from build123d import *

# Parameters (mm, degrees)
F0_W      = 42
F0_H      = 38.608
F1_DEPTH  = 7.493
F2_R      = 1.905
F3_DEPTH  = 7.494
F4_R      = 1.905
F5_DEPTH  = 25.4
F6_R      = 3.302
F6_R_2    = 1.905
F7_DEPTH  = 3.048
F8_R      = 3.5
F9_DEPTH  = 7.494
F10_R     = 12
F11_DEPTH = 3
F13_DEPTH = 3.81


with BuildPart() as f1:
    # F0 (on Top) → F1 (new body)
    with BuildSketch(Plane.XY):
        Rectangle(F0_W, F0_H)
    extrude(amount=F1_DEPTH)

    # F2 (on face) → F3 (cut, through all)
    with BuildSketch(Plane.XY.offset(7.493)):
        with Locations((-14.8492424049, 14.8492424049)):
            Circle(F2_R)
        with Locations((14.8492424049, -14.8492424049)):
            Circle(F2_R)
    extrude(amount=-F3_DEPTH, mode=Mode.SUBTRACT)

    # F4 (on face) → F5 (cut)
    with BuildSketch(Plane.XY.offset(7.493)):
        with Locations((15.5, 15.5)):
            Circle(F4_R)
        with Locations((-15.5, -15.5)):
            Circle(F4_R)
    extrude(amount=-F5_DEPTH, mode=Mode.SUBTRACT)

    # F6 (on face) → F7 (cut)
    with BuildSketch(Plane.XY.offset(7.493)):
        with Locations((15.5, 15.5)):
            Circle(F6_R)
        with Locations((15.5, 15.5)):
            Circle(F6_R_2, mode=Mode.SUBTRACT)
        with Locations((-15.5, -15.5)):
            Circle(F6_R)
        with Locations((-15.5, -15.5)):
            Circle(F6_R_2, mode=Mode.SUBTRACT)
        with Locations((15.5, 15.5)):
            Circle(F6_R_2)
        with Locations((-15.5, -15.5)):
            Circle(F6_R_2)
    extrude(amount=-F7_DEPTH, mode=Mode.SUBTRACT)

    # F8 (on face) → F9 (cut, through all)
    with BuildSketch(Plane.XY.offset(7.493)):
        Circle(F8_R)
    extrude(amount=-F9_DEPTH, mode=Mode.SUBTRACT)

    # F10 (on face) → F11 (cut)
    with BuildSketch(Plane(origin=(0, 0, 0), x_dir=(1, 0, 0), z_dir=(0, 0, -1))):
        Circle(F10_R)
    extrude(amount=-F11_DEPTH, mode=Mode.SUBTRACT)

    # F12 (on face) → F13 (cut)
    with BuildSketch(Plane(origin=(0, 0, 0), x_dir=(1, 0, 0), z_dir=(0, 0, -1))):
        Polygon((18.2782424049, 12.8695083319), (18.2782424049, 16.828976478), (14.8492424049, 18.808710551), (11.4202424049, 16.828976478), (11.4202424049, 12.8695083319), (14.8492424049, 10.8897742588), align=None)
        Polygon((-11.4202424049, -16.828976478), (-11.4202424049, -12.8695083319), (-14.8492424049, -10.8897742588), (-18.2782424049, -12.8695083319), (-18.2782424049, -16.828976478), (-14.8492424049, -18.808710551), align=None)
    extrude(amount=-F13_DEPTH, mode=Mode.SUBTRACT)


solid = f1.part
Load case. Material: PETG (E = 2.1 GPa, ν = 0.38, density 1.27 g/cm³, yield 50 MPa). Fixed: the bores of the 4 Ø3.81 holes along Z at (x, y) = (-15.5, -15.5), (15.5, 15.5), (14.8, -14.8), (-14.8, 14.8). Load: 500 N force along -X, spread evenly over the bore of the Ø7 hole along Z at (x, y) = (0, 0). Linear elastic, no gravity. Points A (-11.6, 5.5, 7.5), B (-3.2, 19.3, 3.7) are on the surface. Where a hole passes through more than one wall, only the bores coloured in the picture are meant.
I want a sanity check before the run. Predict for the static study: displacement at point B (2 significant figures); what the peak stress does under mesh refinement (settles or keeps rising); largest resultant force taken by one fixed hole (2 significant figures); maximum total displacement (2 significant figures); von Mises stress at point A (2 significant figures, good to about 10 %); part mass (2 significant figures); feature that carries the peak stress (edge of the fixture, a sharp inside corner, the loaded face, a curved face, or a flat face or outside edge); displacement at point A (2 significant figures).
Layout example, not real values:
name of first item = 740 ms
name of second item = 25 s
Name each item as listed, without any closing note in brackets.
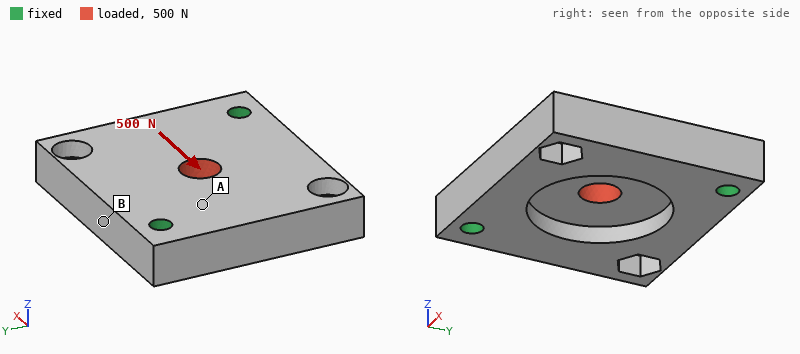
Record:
displacement at point B = 11 µm
what the peak stress does under mesh refinement = keeps rising
largest resultant force taken by one fixed hole = 140 N
maximum total displacement = 37 µm
von Mises stress at point A = 2.6 MPa
part mass = 13 g
feature that carries the peak stress = edge of the fixture
displacement at point A = 20 µm
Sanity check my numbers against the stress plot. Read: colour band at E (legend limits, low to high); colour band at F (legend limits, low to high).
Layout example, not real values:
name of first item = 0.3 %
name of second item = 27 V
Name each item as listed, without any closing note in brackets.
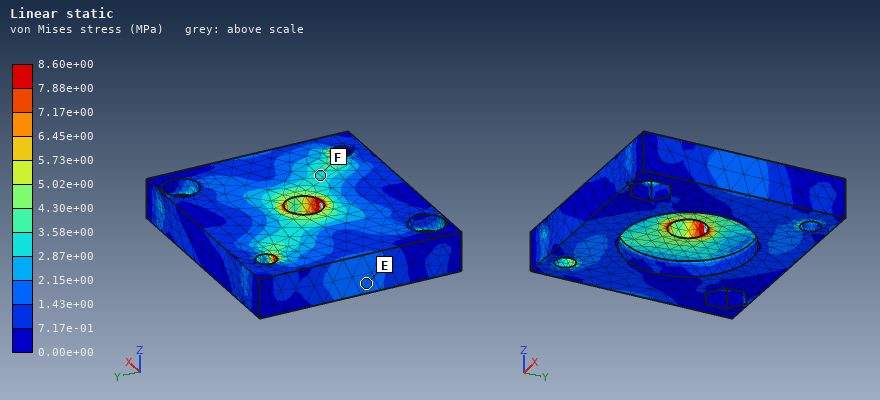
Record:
colour band at E = 1.43e+00 to 2.15e+00 MPa
colour band at F = 2.87e+00 to 3.58e+00 MPa
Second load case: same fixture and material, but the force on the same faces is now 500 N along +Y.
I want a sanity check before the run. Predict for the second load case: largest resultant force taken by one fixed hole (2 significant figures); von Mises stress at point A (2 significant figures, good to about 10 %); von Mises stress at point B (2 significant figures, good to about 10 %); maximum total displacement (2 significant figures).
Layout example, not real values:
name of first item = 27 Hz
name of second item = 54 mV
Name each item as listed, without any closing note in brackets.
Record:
largest resultant force taken by one fixed hole = 140 N
von Mises stress at point A = 2.1 MPa
von Mises stress at point B = 1.8 MPa
maximum total displacement = 38 µm
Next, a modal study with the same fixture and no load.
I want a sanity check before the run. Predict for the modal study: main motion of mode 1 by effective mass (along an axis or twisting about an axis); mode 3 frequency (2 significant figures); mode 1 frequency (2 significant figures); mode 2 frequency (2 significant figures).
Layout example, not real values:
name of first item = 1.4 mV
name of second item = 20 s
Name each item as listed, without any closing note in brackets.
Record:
main motion of mode 1 by effective mass = along Z
mode 3 frequency = 6400 Hz
mode 1 frequency = 5000 Hz
mode 2 frequency = 6400 Hz
